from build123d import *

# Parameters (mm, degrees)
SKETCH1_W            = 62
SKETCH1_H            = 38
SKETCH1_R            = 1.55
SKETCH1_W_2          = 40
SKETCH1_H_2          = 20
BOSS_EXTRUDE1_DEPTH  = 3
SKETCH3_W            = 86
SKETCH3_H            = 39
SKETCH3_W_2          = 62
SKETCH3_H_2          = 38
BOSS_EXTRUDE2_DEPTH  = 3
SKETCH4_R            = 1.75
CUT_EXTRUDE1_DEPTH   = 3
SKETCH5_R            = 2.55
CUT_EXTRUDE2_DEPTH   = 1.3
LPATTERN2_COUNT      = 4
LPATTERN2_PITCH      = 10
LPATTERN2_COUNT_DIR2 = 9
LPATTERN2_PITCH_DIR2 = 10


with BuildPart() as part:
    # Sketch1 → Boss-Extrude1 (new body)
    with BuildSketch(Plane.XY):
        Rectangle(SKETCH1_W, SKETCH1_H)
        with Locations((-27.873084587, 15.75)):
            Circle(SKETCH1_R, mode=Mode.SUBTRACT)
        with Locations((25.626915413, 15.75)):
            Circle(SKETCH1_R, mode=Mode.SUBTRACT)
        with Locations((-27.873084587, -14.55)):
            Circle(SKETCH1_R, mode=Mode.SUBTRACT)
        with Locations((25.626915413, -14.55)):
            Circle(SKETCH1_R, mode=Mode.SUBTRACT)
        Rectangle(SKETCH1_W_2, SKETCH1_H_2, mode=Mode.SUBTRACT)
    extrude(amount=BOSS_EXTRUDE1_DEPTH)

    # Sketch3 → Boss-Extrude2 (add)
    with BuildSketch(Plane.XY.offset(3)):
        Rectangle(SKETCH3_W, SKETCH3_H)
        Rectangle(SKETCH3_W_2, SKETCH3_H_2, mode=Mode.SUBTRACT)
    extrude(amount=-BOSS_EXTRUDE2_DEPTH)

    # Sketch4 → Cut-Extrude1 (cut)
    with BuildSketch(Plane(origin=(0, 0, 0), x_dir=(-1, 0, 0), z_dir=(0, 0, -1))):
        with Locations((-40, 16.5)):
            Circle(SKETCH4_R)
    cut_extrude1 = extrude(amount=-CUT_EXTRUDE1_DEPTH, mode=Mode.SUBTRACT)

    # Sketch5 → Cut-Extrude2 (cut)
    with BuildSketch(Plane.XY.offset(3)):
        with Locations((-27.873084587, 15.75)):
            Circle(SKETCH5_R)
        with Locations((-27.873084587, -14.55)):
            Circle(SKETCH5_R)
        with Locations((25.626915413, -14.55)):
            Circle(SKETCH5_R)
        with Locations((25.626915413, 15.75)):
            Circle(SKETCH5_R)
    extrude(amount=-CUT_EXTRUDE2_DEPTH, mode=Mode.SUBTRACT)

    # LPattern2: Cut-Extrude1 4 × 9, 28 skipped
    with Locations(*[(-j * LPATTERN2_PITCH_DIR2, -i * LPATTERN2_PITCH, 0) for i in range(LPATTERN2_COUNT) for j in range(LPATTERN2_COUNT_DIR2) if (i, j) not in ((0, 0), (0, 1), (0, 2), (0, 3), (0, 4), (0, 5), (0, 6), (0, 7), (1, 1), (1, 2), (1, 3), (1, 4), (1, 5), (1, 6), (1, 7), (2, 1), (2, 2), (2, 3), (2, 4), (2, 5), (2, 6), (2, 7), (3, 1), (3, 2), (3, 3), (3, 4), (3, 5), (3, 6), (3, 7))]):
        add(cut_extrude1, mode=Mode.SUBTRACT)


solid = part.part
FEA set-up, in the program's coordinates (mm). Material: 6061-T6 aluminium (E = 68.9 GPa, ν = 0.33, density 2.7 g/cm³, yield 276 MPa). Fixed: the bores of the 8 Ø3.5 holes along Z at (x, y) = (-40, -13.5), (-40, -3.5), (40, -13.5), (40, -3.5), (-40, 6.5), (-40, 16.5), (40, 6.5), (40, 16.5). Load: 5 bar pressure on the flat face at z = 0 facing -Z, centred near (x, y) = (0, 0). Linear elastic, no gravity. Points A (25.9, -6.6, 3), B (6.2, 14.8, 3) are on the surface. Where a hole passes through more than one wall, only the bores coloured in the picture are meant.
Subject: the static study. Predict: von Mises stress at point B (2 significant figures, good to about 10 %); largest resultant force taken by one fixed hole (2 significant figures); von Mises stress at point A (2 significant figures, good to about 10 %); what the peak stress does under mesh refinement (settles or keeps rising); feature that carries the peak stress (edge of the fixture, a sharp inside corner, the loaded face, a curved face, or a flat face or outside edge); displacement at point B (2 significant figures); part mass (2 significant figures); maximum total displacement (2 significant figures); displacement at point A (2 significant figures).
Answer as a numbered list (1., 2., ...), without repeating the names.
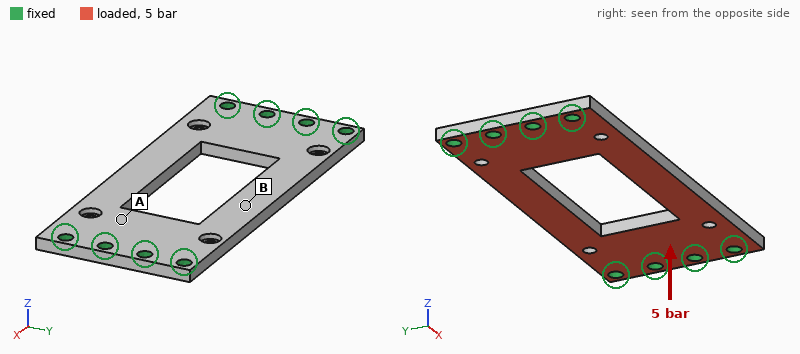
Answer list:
1. 65 MPa
2. 180 N
3. 24 MPa
4. keeps rising
5. edge of the fixture
6. 0.23 mm
7. 20 g
8. 0.25 mm
9. 0.069 mm
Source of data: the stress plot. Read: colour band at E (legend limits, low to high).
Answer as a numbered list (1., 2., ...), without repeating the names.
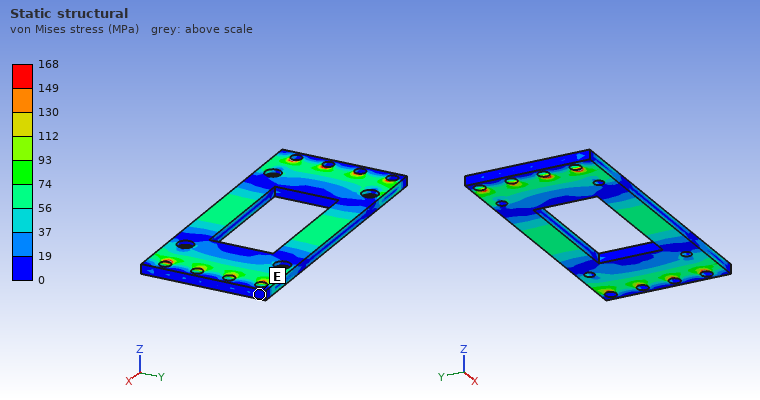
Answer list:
1. 0 to 19 MPa
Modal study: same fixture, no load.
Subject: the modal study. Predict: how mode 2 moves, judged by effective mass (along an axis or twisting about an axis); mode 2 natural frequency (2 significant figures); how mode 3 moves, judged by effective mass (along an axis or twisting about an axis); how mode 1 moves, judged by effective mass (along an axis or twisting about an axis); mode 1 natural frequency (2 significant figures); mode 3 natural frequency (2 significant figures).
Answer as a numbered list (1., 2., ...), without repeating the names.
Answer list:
1. twisting about X
2. 3500 Hz
3. twisting about Y
4. along Z
5. 3000 Hz
6. 7000 Hz
